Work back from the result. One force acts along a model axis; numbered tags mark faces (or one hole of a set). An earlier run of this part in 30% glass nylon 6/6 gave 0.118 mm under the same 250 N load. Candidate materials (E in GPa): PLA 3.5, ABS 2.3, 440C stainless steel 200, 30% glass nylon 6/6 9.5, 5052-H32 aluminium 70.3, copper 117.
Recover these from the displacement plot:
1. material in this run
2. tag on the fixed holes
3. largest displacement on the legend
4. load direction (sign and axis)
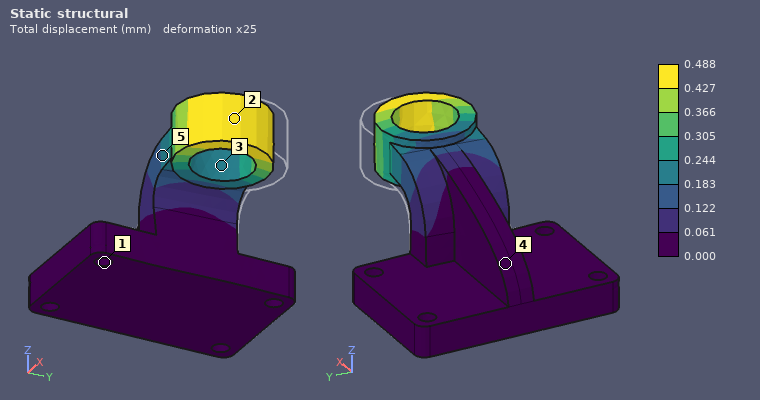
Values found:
ABS
1
0.488 mm
-Y
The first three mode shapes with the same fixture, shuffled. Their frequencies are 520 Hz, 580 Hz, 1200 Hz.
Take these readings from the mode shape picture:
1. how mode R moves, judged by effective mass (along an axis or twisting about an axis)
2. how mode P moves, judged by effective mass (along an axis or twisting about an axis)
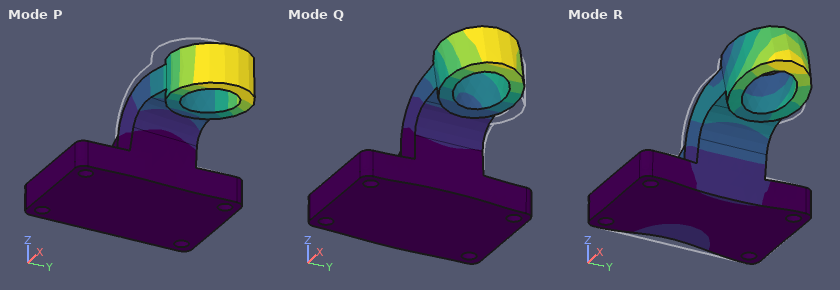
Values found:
along X
along Y
